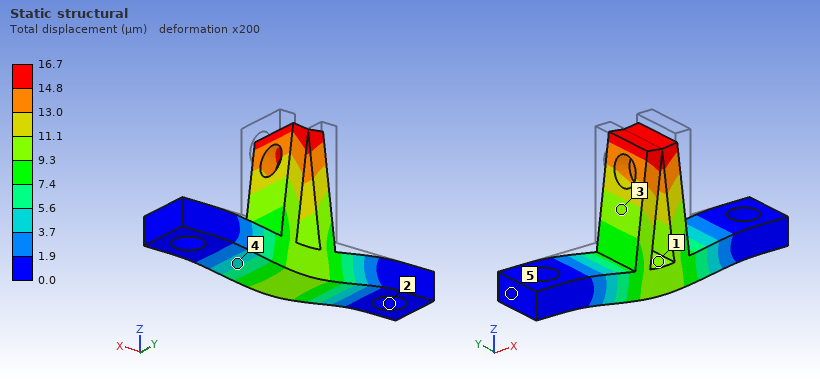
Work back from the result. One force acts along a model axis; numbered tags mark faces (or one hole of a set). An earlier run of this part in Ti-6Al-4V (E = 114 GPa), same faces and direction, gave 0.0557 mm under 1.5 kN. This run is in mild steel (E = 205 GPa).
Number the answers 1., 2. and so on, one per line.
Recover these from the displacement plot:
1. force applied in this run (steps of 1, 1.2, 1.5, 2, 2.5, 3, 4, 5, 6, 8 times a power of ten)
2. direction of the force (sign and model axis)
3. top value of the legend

1. 800 N
2. -Z
3. 16.7 µm
